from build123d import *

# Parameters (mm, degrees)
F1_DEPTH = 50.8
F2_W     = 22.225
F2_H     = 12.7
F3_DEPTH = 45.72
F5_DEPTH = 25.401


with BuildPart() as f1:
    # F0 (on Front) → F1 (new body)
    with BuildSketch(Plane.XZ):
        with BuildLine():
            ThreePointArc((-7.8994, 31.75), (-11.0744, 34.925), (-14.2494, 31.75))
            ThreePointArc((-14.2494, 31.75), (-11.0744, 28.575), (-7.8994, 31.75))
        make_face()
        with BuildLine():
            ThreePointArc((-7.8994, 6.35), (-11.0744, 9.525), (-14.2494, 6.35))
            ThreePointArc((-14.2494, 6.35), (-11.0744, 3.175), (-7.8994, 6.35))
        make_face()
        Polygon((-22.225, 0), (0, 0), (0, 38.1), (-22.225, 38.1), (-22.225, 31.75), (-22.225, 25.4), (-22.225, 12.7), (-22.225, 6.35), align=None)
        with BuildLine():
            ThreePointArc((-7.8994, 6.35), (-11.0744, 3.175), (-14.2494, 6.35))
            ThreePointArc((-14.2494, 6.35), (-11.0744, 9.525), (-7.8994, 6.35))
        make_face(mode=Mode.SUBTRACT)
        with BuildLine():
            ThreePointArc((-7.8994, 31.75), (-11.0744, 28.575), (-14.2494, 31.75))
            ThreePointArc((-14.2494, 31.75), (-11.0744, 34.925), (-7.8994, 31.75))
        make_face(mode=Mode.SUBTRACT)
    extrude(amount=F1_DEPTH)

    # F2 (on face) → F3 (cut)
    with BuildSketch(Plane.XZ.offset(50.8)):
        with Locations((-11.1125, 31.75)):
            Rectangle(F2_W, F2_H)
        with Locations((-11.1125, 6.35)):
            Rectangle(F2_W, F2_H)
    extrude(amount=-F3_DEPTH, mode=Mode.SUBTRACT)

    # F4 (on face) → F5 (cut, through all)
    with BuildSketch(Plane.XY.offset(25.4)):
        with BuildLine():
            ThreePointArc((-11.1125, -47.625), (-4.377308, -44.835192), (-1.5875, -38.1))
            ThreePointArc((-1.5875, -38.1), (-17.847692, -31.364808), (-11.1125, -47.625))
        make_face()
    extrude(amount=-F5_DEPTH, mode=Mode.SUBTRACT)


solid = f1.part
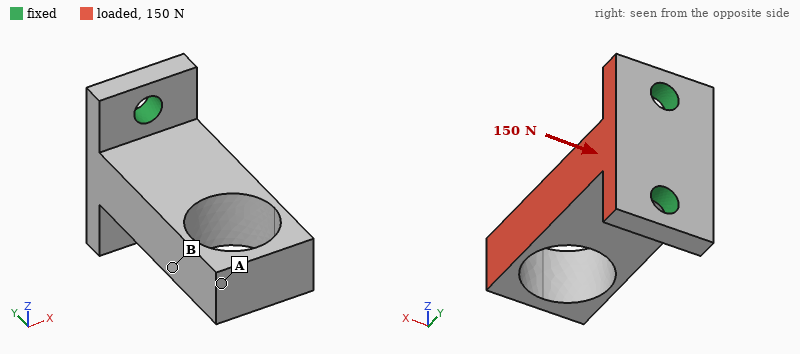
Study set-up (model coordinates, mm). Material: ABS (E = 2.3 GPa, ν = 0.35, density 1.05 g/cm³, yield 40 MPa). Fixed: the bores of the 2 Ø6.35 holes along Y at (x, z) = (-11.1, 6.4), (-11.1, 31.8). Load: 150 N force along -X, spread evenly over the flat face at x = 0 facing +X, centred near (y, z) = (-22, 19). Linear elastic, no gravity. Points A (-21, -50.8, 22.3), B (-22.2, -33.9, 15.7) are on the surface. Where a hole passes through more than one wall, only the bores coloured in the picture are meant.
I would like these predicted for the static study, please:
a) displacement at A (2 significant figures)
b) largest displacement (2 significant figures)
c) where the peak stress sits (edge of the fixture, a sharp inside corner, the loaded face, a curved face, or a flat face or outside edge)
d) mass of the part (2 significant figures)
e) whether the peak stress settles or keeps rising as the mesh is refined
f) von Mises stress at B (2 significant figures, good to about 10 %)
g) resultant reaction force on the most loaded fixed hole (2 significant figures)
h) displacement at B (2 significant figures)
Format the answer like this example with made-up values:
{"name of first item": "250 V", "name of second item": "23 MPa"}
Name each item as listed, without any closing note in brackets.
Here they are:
{"displacement at A": "0.62 mm", "largest displacement": "0.62 mm", "where the peak stress sits": "edge of the fixture", "mass of the part": "14 g", "whether the peak stress settles or keeps rising as the mesh is refined": "keeps rising", "von Mises stress at B": "4.5 MPa", "resultant reaction force on the most loaded fixed hole": "75 N", "displacement at B": "0.35 mm"}
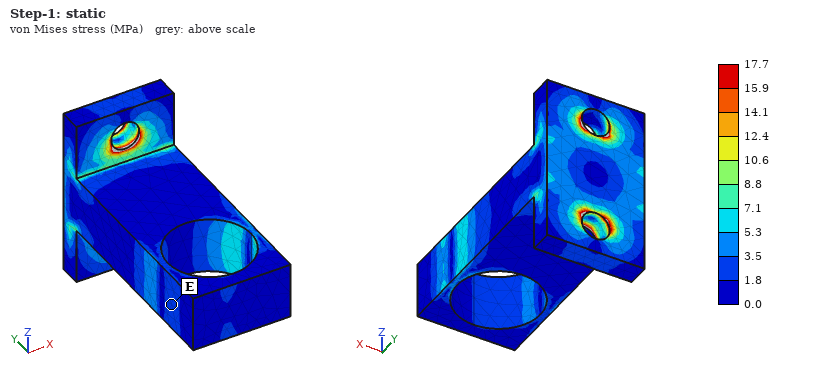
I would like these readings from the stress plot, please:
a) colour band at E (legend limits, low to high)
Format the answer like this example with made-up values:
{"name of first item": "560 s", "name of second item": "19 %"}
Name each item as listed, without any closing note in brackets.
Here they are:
{"colour band at E": "1.8 to 3.5 MPa"}
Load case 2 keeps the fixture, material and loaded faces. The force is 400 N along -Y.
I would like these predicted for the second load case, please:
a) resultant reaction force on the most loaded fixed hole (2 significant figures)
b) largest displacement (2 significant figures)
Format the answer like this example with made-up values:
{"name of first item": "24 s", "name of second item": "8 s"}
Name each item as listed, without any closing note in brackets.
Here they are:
{"resultant reaction force on the most loaded fixed hole": "210 N", "largest displacement": "0.77 mm"}
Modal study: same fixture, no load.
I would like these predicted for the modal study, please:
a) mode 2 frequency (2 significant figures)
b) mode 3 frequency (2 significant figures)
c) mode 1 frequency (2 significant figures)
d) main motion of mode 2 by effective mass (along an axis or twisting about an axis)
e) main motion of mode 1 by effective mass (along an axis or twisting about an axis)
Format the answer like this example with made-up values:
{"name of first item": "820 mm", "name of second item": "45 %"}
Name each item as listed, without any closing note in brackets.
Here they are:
{"mode 2 frequency": "1300 Hz", "mode 3 frequency": "3200 Hz", "mode 1 frequency": "950 Hz", "main motion of mode 2 by effective mass": "along Z", "main motion of mode 1 by effective mass": "along X"}
